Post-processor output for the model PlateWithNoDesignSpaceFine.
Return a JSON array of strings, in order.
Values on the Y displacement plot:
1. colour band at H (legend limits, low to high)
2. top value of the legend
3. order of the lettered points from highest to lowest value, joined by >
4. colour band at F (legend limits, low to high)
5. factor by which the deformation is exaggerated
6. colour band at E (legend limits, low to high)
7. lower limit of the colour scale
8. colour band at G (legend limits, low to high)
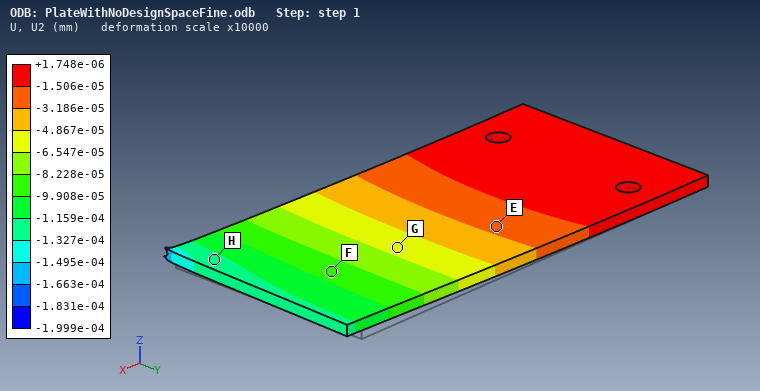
["-1.327e-04 to -1.159e-04 mm", "+1.748e-06 mm", "E > G > F > H", "-9.908e-05 to -8.228e-05 mm", "10000", "-3.186e-05 to -1.506e-05 mm", "-1.999e-04 mm", "-6.547e-05 to -4.867e-05 mm"]
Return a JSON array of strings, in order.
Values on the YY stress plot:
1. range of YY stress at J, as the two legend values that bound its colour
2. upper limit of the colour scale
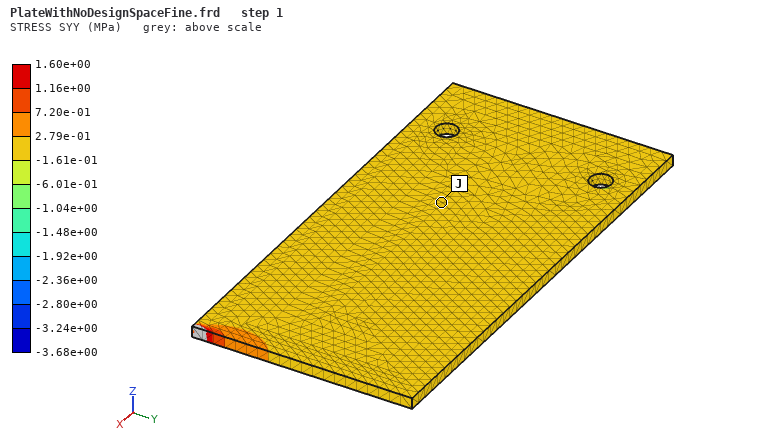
["-1.61e-01 to 2.79e-01 MPa", "1.60e+00 MPa"]
